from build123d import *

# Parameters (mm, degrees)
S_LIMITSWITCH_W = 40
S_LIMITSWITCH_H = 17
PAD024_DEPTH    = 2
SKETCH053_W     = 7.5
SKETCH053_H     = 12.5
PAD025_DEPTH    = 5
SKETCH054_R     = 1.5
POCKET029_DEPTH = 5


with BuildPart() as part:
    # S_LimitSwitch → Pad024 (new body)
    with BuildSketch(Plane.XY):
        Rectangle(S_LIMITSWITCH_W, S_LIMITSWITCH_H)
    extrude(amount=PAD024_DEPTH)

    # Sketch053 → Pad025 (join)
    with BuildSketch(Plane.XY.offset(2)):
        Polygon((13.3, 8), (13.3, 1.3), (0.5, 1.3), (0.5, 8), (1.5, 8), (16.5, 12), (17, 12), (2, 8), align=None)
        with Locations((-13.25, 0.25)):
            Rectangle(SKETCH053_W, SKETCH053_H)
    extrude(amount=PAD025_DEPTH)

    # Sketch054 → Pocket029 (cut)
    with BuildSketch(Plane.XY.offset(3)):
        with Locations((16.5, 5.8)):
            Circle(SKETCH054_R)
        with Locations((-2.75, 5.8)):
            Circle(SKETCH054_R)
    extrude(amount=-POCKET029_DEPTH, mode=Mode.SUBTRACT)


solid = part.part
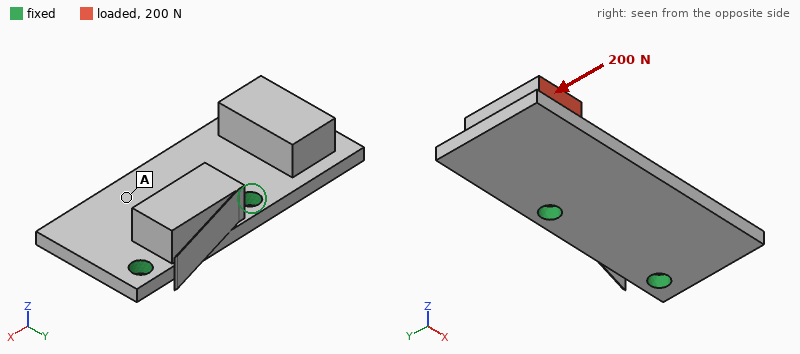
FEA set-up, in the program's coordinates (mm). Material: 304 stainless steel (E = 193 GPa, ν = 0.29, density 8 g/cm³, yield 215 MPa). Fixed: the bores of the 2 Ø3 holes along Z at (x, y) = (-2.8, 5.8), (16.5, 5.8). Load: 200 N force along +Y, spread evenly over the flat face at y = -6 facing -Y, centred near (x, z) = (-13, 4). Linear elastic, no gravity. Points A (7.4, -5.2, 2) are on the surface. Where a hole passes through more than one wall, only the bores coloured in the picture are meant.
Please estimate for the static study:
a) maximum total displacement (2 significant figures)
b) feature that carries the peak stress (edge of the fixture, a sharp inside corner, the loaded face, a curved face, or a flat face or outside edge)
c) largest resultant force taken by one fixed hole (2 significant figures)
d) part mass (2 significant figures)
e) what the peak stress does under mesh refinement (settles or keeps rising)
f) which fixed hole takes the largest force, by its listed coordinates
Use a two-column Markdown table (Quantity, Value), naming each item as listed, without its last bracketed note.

| Quantity | Value |
|---|---|
| maximum total displacement | 24 µm |
| feature that carries the peak stress | edge of the fixture |
| largest resultant force taken by one fixed hole | 290 N |
| part mass | 18 g |
| what the peak stress does under mesh refinement | keeps rising |
| which fixed hole takes the largest force, by its listed coordinates | (-2.8, 5.8) |
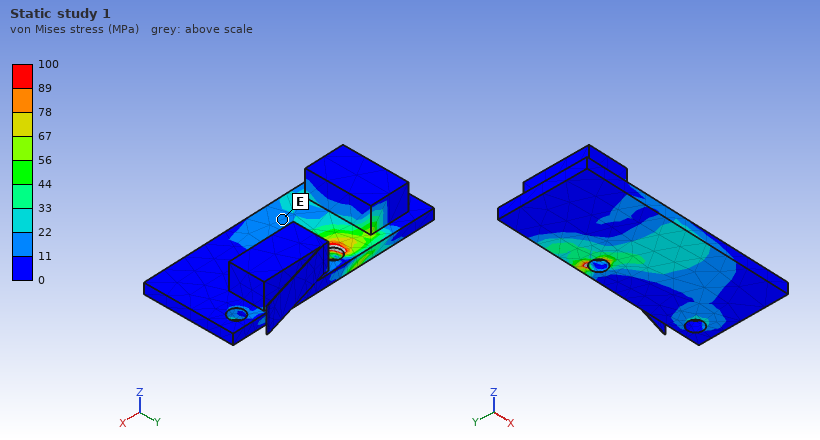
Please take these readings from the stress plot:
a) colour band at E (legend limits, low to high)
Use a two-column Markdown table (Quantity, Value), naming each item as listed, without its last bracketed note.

| Quantity | Value |
|---|---|
| colour band at E | 11 to 22 MPa |
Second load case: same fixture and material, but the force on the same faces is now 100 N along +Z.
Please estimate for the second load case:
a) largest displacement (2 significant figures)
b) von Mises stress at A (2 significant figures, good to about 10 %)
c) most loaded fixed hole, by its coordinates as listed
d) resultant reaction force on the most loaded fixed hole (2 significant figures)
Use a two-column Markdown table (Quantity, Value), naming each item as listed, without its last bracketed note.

| Quantity | Value |
|---|---|
| largest displacement | 76 µm |
| von Mises stress at A | 24 MPa |
| most loaded fixed hole, by its coordinates as listed | (-2.8, 5.8) |
| resultant reaction force on the most loaded fixed hole | 130 N |
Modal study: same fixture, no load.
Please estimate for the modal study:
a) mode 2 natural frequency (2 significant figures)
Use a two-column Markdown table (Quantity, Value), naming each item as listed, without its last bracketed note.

| Quantity | Value |
|---|---|
| mode 2 natural frequency | 3200 Hz |
